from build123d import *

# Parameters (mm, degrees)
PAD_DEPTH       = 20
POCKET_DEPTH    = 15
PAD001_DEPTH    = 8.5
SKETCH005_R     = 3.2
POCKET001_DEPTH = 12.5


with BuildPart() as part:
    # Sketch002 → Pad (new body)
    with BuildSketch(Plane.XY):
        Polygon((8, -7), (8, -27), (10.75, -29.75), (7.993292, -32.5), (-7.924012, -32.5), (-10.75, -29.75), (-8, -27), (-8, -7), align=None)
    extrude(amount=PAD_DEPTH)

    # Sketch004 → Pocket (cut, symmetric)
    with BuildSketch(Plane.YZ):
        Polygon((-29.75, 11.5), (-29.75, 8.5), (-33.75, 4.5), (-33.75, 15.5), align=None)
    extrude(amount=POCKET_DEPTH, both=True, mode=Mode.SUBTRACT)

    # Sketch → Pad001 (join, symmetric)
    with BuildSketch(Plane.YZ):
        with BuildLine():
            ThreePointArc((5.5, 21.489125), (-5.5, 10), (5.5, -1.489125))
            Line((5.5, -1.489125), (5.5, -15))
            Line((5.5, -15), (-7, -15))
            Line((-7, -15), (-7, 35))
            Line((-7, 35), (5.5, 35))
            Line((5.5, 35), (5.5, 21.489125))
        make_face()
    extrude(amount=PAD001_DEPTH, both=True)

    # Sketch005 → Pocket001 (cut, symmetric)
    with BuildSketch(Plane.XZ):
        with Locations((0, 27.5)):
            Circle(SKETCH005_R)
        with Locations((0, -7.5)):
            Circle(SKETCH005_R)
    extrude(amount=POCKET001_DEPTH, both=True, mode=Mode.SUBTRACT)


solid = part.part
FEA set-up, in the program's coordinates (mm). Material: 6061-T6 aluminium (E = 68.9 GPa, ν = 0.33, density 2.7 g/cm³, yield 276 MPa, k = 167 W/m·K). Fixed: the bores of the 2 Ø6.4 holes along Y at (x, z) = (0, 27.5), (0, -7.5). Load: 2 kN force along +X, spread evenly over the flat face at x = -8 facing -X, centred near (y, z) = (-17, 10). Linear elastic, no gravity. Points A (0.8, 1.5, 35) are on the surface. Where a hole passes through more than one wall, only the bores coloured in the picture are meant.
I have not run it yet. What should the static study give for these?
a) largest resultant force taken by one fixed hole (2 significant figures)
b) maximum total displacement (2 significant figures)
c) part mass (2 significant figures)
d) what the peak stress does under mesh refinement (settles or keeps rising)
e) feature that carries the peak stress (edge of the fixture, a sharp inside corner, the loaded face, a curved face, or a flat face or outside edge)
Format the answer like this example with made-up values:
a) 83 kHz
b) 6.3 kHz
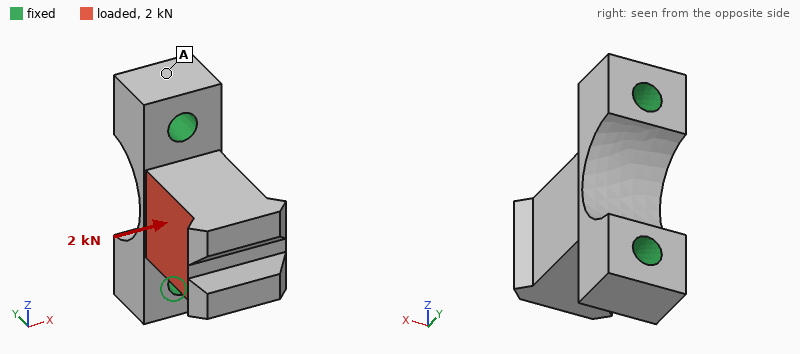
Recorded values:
a) 1.0 kN
b) 62 µm
c) 40 g
d) keeps rising
e) edge of the fixture
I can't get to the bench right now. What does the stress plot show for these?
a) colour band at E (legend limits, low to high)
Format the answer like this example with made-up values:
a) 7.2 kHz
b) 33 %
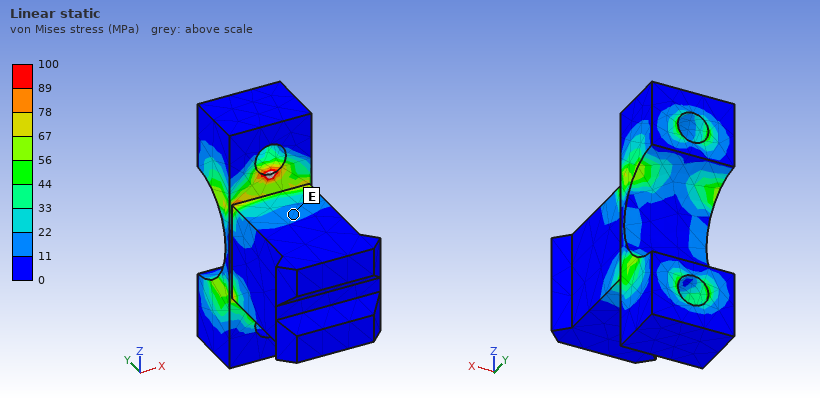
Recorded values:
a) 11 to 22 MPa
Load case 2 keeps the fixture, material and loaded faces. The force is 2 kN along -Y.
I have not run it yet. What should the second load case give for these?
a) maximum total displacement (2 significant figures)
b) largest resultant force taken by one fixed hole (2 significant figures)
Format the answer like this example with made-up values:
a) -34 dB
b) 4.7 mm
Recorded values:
a) 38 µm
b) 1.2 kN
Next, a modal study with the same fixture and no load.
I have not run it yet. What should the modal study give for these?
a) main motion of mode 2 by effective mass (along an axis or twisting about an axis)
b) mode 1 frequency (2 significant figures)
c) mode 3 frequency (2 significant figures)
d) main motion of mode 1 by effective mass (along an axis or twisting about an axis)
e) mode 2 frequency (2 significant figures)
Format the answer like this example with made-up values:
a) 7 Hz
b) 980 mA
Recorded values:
a) along Z
b) 6600 Hz
c) 21 kHz
d) along X
e) 12 kHz
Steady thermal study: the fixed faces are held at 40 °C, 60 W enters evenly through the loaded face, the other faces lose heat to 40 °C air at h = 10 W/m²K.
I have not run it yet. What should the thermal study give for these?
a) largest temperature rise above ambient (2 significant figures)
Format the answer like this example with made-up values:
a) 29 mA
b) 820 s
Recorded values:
a) 31 K
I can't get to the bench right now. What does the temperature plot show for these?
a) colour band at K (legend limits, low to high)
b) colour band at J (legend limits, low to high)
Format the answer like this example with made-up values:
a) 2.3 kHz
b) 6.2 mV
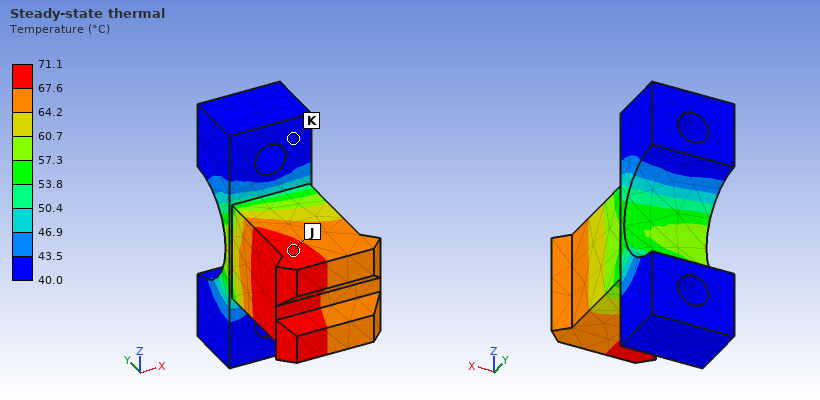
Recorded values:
a) 40.0 to 43.5 °C
b) 67.6 to 71.1 °C
